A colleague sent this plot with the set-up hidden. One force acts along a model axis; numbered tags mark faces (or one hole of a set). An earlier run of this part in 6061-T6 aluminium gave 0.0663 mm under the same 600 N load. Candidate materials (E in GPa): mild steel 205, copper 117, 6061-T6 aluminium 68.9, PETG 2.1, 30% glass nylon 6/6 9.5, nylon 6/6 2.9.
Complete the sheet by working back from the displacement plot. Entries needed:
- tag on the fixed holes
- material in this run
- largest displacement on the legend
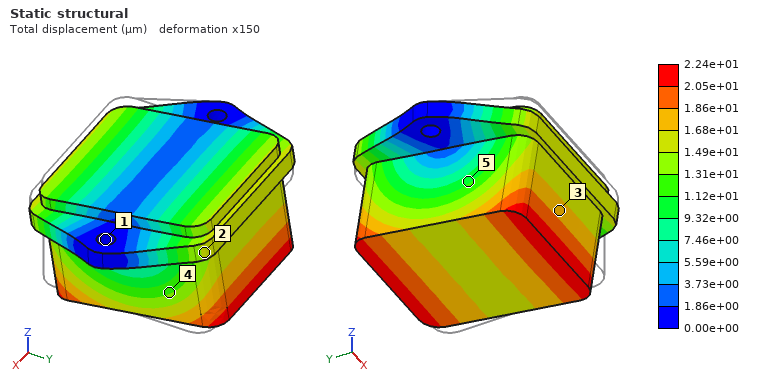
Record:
1
mild steel
2.24e+01 µm
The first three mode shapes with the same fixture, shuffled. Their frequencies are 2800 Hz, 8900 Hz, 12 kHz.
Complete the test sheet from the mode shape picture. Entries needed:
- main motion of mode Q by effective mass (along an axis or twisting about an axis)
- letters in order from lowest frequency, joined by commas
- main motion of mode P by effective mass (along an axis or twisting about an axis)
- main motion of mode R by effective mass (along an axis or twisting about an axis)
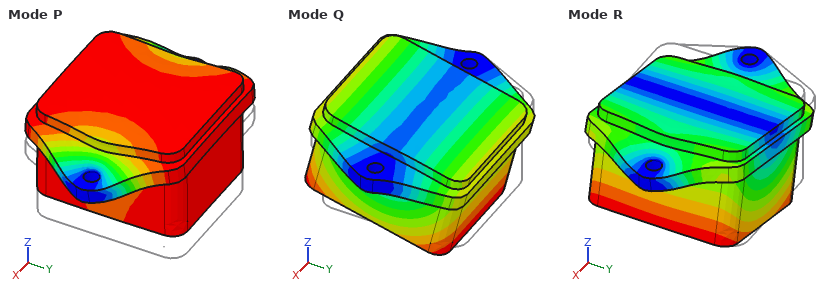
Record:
along Y
Q, P, R
along Z
along X
